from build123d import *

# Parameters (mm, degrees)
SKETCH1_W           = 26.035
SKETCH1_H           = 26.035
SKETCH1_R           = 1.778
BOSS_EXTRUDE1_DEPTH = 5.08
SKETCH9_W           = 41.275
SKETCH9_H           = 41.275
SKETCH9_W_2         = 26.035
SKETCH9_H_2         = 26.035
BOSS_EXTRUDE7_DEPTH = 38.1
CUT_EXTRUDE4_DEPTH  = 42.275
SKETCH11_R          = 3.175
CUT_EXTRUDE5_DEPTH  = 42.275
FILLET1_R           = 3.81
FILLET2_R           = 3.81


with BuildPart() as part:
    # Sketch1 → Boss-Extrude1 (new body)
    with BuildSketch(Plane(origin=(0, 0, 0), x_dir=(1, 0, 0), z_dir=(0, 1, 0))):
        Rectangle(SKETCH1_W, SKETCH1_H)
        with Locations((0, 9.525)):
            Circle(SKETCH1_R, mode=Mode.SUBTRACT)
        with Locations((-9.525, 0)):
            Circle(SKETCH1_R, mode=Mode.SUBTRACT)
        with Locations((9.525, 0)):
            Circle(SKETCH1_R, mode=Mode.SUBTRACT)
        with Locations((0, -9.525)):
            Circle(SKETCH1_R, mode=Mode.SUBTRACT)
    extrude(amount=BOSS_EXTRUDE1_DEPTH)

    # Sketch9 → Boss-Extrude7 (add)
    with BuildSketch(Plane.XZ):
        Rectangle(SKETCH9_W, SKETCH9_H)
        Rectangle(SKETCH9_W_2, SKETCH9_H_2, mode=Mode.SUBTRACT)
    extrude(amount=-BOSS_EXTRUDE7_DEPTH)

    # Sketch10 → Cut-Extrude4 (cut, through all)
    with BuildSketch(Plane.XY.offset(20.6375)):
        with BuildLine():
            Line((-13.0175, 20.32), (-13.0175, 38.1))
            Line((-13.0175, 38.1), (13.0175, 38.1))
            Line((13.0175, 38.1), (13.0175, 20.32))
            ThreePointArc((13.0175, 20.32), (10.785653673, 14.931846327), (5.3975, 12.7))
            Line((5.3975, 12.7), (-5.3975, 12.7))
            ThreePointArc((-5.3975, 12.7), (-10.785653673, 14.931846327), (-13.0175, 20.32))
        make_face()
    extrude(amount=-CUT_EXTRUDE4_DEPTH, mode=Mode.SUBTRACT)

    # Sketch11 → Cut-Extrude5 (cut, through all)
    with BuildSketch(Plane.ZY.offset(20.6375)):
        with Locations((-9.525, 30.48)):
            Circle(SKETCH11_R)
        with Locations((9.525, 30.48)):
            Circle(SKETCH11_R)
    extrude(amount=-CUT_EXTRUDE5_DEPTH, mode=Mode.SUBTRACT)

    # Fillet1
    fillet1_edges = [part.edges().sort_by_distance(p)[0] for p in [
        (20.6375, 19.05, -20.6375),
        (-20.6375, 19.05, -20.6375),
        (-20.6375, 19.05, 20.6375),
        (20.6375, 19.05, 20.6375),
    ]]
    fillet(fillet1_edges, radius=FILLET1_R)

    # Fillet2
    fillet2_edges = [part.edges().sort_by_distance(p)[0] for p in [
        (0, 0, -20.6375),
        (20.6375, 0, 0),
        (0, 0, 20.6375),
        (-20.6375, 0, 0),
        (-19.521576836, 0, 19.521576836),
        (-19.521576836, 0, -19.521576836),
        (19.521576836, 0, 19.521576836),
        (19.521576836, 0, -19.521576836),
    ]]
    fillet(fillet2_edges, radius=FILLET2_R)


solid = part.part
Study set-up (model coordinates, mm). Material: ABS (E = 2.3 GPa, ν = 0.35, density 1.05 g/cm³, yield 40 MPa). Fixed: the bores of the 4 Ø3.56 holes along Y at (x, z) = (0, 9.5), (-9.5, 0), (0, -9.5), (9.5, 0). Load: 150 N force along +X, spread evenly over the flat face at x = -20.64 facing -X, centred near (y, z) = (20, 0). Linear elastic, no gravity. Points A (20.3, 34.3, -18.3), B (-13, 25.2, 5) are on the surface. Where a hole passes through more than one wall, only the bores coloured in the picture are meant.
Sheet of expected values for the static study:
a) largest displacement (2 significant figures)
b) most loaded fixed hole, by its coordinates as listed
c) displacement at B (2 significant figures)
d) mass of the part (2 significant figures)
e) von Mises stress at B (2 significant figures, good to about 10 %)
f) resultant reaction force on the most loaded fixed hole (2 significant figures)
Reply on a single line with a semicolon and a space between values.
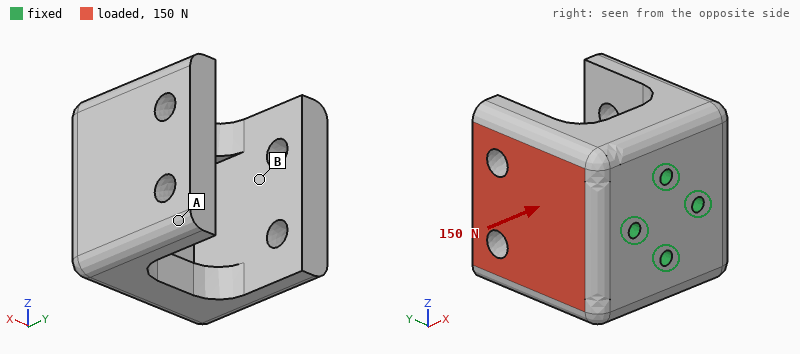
0.28 mm; (-9.5, 0); 0.15 mm; 32 g; 1.5 MPa; 120 N
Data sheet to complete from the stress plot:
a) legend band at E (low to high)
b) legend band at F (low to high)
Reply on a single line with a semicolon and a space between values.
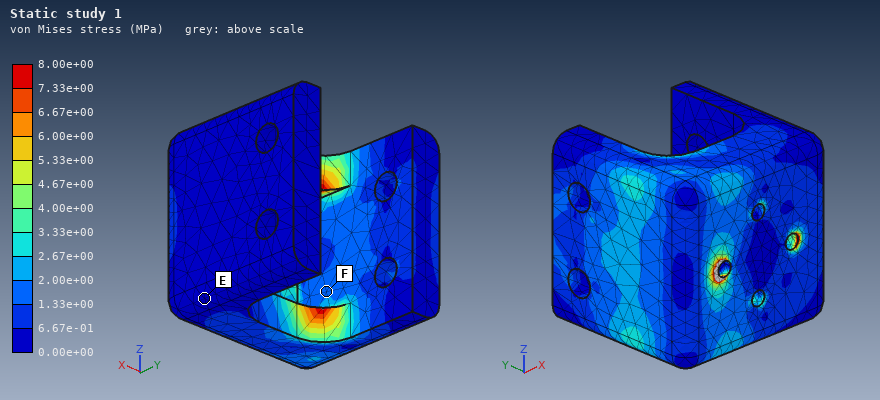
0.00e+00 to 6.67e-01 MPa; 1.33e+00 to 2.00e+00 MPa
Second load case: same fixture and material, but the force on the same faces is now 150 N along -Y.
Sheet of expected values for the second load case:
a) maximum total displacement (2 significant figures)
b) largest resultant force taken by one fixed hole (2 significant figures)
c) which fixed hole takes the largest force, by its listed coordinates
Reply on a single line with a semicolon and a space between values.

0.17 mm; 170 N; (-9.5, 0)
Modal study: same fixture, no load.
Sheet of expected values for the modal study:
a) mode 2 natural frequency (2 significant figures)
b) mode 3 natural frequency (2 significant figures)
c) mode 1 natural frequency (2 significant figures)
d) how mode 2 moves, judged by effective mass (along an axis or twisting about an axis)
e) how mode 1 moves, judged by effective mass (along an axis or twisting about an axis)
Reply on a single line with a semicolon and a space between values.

1500 Hz; 1600 Hz; 1300 Hz; along Z; along X
